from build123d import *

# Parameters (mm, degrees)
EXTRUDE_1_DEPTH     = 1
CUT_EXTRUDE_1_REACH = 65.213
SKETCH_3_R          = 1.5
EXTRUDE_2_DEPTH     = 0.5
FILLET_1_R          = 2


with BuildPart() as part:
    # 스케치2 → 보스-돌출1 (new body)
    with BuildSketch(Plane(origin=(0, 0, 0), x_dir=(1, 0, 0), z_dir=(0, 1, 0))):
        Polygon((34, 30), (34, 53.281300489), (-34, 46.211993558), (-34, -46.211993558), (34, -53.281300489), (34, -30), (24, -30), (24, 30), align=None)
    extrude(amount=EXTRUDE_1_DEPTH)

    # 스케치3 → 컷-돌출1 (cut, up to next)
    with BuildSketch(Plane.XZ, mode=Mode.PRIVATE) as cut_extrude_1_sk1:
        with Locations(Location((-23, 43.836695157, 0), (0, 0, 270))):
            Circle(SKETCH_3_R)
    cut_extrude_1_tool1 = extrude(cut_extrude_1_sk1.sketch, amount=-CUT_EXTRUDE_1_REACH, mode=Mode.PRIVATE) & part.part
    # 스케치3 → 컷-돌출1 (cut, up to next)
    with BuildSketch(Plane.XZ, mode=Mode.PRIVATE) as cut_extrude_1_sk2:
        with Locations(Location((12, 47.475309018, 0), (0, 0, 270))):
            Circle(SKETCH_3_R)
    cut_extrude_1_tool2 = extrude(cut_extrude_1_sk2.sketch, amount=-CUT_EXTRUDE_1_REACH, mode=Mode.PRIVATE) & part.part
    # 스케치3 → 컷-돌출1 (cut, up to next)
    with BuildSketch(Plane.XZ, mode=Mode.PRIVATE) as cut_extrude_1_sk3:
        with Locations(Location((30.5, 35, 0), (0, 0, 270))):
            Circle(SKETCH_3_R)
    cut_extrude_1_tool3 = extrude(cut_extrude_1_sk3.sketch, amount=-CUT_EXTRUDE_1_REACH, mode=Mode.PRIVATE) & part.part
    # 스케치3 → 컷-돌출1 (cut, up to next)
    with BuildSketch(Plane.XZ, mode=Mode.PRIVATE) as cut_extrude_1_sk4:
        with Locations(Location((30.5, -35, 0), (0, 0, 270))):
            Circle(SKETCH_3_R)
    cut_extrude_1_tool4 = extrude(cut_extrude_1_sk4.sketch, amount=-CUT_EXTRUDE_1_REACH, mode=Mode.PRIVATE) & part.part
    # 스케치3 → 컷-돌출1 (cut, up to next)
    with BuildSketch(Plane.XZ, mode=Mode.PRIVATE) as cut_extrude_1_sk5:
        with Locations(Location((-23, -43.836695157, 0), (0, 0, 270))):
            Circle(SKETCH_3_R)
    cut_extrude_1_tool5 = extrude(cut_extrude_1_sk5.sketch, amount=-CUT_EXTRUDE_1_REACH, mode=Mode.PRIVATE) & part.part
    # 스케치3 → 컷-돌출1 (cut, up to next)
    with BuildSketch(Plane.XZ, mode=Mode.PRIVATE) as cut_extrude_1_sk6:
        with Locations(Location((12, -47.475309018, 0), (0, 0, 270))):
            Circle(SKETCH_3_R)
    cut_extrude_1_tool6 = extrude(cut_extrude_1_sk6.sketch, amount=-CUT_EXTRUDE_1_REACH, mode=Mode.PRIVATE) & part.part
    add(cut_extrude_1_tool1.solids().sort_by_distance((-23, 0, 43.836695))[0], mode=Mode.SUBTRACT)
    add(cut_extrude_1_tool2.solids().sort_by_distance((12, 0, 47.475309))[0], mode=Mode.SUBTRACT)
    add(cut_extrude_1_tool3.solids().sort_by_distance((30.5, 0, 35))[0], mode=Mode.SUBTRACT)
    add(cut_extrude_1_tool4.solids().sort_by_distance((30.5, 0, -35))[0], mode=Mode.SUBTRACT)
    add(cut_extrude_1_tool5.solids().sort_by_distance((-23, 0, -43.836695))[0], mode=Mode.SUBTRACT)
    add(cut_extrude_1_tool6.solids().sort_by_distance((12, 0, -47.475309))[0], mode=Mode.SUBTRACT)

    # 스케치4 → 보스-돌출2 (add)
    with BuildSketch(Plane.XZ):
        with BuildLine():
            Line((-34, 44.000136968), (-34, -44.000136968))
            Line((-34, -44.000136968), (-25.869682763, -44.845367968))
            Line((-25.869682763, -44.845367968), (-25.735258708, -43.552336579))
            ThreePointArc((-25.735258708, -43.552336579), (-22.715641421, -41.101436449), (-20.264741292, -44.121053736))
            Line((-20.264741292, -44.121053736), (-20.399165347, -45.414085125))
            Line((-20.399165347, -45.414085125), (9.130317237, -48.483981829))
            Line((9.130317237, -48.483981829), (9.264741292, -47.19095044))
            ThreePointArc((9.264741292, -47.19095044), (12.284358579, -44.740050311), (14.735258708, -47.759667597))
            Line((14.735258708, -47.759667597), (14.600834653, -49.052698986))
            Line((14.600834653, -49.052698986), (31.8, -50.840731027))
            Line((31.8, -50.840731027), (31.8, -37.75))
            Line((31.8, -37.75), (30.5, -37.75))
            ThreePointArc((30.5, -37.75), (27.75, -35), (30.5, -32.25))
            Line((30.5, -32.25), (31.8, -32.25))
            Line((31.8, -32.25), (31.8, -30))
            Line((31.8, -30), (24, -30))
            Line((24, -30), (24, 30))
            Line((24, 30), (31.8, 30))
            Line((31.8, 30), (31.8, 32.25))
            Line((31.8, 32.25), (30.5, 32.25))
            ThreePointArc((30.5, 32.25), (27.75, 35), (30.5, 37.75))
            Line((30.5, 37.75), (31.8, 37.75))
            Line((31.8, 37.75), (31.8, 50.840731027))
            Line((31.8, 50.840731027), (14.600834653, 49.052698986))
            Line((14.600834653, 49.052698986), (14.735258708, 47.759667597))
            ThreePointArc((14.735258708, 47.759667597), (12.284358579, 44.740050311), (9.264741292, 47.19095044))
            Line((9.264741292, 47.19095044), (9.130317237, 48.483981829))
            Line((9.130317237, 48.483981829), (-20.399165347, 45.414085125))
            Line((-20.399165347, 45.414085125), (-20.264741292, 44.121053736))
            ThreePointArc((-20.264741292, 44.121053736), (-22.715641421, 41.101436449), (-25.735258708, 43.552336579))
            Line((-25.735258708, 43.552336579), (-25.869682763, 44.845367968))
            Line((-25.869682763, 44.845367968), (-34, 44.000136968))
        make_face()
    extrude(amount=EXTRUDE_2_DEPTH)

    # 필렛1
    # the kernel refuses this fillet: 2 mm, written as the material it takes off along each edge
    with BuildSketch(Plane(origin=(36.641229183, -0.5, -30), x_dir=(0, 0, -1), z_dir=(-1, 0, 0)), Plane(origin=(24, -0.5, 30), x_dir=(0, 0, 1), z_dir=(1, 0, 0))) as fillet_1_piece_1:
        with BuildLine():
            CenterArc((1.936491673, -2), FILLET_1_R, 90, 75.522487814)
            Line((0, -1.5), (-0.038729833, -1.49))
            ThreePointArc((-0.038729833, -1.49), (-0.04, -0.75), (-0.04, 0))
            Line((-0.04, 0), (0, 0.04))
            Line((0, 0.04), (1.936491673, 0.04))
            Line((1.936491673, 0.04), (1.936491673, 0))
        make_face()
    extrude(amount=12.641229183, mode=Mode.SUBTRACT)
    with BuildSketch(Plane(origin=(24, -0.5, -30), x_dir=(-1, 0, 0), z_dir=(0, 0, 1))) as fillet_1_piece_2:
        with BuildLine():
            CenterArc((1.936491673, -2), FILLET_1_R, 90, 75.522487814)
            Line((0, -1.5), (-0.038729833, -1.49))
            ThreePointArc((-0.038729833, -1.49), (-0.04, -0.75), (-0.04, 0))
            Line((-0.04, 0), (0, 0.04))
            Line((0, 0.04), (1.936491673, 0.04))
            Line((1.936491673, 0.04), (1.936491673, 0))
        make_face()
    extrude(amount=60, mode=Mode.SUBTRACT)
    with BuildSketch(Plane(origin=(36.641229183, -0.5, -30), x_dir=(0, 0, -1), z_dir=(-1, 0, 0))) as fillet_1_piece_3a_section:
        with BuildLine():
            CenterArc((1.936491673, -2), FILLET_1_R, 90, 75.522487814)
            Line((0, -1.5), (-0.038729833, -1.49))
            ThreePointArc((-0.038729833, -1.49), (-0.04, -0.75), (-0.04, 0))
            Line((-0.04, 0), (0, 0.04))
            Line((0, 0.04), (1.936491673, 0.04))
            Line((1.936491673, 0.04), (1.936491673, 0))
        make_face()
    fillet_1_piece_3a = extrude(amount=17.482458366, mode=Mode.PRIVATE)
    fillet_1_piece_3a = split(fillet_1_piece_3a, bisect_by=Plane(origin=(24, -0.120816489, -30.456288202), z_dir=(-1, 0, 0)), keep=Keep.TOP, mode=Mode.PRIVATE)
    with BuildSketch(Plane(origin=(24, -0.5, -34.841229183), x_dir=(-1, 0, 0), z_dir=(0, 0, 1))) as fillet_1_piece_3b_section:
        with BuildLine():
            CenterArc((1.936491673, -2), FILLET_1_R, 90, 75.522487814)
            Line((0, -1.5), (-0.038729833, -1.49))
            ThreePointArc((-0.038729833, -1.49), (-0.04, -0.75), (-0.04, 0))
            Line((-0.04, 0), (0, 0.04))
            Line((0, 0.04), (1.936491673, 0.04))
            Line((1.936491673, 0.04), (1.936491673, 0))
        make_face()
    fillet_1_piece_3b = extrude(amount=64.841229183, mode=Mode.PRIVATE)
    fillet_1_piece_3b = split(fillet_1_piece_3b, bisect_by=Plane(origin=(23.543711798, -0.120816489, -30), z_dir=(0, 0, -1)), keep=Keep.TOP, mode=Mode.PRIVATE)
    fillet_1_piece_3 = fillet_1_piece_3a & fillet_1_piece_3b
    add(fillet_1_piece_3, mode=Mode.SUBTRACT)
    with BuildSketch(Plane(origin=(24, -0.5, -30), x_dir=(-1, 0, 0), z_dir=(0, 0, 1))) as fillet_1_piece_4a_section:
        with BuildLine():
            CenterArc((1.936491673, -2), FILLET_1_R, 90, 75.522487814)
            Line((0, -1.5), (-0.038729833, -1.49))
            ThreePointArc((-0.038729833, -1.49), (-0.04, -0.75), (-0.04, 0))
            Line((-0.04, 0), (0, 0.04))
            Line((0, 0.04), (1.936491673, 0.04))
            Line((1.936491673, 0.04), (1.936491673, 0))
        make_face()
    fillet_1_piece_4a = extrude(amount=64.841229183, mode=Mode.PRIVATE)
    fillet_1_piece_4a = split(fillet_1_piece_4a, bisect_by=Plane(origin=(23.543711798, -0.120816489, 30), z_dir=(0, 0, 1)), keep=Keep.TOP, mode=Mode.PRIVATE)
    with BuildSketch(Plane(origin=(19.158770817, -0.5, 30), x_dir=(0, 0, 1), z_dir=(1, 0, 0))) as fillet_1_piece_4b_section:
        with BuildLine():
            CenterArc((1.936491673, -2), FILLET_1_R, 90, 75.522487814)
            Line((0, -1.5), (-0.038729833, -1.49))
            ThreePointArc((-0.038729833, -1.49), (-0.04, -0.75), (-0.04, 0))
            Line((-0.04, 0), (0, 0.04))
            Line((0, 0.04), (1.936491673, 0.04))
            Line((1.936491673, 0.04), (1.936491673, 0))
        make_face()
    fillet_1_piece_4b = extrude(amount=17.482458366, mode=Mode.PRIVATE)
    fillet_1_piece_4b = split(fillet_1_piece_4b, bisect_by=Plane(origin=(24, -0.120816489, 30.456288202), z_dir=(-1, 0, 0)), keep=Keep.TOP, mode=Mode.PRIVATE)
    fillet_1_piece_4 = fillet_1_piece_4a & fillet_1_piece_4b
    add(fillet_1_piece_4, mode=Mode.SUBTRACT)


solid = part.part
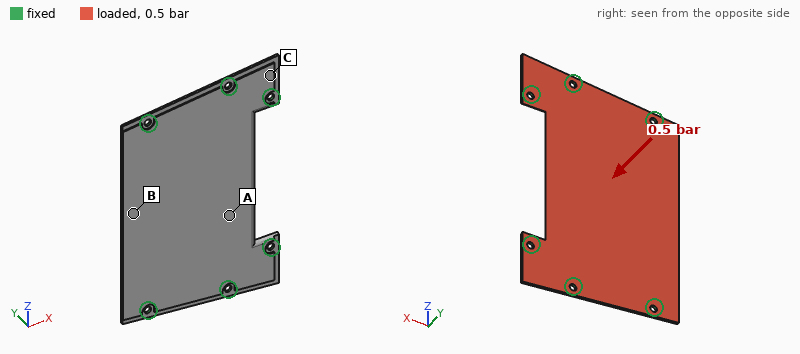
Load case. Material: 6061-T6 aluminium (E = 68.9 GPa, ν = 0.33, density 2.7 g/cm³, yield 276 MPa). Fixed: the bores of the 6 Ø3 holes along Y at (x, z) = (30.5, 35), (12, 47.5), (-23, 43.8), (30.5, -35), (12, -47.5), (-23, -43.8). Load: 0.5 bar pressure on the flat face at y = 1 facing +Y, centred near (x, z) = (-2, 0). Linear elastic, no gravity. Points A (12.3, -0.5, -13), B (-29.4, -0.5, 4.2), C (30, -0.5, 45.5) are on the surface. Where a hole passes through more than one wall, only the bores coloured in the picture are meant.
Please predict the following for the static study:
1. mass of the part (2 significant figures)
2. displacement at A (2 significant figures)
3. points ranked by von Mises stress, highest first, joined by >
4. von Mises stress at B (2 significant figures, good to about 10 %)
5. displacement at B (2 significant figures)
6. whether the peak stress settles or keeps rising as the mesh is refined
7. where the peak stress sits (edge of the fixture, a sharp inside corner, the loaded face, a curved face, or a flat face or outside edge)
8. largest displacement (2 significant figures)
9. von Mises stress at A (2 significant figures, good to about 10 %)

24 g
0.38 mm
B > A > C
53 MPa
0.56 mm
keeps rising
edge of the fixture
0.59 mm
34 MPa
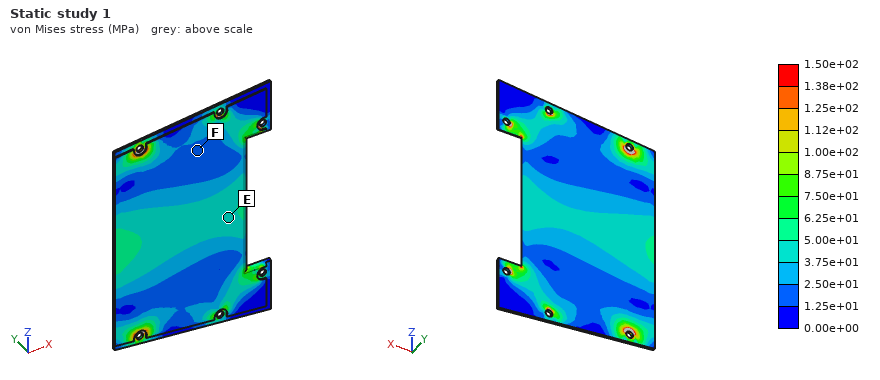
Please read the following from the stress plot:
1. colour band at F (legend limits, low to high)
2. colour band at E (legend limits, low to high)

1.25e+01 to 2.50e+01 MPa
3.75e+01 to 5.00e+01 MPa
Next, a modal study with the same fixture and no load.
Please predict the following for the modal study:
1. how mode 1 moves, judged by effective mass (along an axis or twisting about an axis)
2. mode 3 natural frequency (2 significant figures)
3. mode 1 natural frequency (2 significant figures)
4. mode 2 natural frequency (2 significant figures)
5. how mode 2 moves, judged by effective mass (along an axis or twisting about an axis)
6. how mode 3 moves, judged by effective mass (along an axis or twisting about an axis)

along Y
2400 Hz
890 Hz
1500 Hz
twisting about Z
twisting about X
